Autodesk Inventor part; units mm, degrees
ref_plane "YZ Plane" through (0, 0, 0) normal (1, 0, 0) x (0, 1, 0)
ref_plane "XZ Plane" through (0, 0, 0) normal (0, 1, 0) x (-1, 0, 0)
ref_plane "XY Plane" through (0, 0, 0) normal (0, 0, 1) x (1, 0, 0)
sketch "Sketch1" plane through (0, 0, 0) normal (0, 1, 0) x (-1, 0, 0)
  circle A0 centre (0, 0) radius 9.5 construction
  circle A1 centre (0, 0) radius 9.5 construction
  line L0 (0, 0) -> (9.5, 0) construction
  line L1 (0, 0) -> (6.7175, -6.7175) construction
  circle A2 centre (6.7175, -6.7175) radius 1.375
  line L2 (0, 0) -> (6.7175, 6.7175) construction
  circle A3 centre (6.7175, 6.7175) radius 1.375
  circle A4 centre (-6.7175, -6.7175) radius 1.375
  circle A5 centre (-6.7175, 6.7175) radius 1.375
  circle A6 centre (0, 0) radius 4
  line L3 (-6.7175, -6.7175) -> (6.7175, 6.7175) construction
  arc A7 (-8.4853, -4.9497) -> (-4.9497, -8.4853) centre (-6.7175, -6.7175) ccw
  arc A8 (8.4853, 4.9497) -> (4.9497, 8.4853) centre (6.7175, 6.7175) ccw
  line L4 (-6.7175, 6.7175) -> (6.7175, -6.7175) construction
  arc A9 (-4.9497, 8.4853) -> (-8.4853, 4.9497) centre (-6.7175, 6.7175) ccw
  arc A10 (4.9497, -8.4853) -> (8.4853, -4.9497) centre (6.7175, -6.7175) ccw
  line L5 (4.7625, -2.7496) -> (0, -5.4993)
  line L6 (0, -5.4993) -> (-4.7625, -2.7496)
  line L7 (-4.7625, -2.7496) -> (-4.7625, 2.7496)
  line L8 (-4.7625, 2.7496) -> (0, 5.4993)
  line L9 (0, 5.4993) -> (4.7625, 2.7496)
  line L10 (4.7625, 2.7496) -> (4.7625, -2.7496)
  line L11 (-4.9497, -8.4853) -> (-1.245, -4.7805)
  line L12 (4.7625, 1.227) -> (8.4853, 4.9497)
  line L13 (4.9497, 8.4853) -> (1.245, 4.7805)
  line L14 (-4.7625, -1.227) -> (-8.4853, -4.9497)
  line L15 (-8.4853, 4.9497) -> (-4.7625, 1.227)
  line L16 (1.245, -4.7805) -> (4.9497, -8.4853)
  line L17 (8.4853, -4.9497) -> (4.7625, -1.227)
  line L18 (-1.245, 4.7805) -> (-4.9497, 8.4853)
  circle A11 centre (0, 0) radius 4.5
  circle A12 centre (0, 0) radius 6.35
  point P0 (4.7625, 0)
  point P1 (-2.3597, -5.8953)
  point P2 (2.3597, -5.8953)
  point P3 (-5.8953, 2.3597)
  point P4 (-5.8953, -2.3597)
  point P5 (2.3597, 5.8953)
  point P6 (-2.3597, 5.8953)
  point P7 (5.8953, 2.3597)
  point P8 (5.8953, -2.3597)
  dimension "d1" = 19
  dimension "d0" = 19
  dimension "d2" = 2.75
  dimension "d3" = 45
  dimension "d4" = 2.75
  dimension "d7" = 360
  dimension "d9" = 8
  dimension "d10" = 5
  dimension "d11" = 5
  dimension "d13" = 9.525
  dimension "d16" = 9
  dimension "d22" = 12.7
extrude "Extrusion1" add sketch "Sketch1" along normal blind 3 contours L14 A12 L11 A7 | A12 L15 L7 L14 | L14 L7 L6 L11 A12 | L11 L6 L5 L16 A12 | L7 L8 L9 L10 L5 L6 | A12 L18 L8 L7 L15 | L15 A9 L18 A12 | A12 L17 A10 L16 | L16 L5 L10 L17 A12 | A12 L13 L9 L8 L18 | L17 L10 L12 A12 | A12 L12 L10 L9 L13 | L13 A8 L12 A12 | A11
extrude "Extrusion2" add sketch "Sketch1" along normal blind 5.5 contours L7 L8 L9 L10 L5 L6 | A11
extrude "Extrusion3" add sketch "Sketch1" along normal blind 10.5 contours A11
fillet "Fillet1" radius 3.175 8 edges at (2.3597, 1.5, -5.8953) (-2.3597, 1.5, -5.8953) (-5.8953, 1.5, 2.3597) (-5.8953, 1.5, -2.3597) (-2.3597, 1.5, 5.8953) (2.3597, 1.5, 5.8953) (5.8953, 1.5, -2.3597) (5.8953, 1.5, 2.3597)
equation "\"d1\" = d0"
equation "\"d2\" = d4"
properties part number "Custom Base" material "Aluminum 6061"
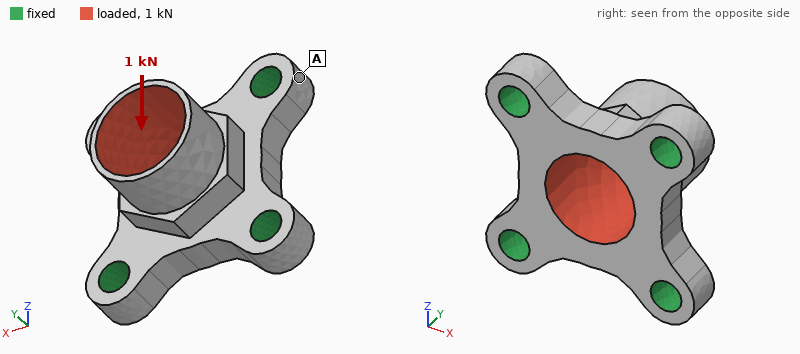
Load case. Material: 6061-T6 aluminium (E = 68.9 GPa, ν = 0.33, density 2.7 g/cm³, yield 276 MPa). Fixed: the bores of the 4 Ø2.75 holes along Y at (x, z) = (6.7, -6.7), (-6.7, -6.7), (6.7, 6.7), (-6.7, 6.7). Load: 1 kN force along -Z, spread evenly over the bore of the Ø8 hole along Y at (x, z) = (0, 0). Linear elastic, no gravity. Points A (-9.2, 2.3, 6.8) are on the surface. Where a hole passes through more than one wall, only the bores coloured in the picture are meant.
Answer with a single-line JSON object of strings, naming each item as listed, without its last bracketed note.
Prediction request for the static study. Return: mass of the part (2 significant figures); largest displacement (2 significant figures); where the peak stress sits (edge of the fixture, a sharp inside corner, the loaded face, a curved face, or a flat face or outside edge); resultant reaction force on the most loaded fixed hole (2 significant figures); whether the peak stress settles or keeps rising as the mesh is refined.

{"mass of the part": "1.7 g", "largest displacement": "26 µm", "where the peak stress sits": "edge of the fixture", "resultant reaction force on the most loaded fixed hole": "330 N", "whether the peak stress settles or keeps rising as the mesh is refined": "keeps rising"}
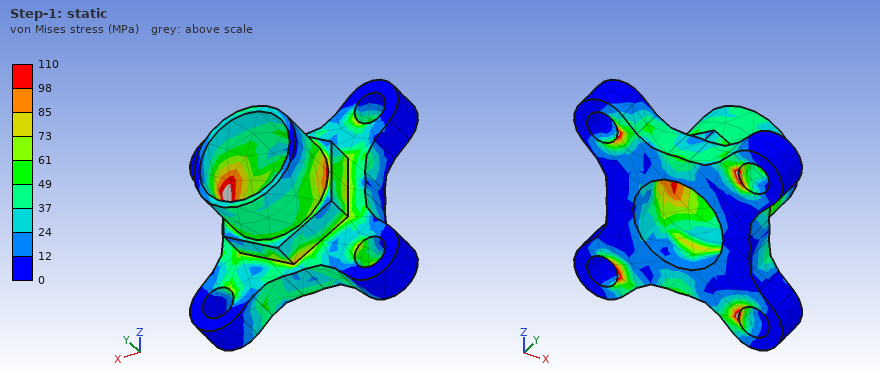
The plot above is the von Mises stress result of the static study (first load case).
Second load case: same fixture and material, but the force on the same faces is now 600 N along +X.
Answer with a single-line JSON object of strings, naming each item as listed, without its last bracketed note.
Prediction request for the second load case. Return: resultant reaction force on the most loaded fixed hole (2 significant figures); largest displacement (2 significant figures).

{"resultant reaction force on the most loaded fixed hole": "200 N", "largest displacement": "15 µm"}
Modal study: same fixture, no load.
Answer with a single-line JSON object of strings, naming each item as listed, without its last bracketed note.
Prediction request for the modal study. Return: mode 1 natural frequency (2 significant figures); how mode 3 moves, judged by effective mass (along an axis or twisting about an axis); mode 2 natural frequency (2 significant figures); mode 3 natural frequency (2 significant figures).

{"mode 1 natural frequency": "42 kHz", "how mode 3 moves, judged by effective mass": "along Z", "mode 2 natural frequency": "47 kHz", "mode 3 natural frequency": "54 kHz"}
